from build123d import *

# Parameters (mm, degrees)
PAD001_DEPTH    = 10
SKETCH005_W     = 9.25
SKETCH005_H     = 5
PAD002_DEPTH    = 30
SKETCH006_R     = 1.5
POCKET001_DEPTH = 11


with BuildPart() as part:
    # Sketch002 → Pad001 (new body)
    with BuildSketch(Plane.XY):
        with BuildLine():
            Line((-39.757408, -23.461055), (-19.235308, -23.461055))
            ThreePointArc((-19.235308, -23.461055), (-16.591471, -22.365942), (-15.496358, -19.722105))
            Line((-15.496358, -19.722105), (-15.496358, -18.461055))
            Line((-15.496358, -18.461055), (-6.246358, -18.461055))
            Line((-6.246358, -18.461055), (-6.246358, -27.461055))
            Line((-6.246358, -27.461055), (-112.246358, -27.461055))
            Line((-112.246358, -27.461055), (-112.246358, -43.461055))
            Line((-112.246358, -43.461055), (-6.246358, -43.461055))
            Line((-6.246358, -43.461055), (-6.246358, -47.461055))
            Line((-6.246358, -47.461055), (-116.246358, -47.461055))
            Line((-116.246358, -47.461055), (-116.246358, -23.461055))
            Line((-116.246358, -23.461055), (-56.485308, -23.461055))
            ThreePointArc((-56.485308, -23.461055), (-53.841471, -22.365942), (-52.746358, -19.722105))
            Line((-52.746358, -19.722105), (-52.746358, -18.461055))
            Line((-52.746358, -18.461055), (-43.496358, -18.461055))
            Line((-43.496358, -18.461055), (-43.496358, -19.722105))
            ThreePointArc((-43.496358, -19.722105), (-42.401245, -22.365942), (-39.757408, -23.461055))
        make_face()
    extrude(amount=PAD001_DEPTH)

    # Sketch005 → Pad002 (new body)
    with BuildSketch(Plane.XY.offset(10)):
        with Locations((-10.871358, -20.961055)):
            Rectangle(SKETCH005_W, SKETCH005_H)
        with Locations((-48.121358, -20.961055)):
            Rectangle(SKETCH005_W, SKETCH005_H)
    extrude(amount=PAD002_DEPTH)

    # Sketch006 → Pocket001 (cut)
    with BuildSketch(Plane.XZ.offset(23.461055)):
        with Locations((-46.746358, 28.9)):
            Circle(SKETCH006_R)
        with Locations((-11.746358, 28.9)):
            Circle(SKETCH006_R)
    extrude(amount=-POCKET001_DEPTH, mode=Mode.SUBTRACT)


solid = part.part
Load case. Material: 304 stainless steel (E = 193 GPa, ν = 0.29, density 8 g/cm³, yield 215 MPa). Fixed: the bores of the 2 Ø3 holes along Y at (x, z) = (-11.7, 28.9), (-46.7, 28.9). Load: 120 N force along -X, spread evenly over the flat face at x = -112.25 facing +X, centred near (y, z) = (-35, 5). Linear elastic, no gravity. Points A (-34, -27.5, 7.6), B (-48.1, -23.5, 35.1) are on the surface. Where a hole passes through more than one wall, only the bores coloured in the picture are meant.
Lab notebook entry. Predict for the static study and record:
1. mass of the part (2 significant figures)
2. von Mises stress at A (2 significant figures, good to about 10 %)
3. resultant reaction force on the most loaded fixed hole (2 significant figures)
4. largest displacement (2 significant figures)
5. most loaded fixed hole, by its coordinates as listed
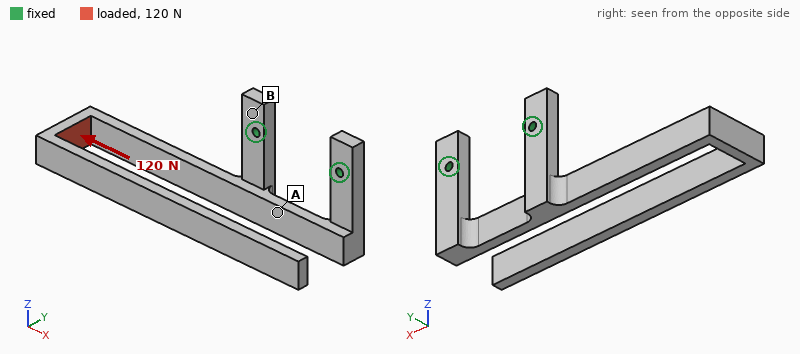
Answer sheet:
110 g
17 MPa
95 N
0.66 mm
(-11.7, 28.9)
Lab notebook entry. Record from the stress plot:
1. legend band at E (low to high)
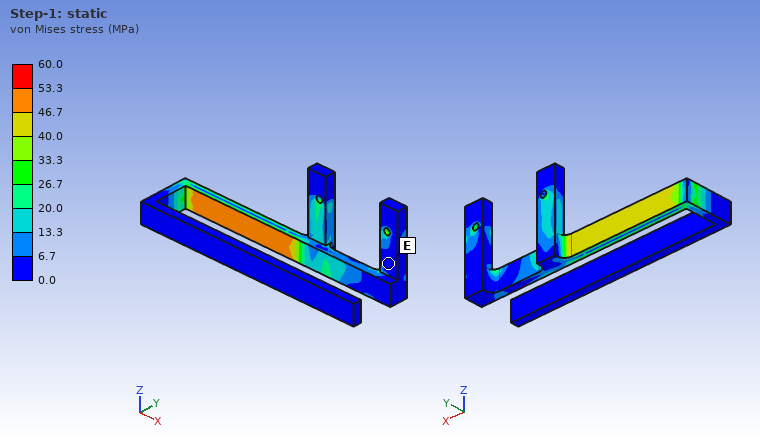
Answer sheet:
0.0 to 6.7 MPa
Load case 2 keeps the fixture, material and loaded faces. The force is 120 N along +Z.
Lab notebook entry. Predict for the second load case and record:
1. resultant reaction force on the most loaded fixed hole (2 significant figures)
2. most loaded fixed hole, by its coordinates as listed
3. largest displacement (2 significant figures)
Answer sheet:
300 N
(-46.7, 28.9)
0.41 mm
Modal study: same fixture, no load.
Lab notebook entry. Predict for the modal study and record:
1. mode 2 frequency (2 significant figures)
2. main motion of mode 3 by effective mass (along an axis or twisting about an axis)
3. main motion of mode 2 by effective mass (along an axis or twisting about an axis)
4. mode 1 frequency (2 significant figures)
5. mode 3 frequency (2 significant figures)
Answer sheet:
260 Hz
along Y
along Z
160 Hz
340 Hz
